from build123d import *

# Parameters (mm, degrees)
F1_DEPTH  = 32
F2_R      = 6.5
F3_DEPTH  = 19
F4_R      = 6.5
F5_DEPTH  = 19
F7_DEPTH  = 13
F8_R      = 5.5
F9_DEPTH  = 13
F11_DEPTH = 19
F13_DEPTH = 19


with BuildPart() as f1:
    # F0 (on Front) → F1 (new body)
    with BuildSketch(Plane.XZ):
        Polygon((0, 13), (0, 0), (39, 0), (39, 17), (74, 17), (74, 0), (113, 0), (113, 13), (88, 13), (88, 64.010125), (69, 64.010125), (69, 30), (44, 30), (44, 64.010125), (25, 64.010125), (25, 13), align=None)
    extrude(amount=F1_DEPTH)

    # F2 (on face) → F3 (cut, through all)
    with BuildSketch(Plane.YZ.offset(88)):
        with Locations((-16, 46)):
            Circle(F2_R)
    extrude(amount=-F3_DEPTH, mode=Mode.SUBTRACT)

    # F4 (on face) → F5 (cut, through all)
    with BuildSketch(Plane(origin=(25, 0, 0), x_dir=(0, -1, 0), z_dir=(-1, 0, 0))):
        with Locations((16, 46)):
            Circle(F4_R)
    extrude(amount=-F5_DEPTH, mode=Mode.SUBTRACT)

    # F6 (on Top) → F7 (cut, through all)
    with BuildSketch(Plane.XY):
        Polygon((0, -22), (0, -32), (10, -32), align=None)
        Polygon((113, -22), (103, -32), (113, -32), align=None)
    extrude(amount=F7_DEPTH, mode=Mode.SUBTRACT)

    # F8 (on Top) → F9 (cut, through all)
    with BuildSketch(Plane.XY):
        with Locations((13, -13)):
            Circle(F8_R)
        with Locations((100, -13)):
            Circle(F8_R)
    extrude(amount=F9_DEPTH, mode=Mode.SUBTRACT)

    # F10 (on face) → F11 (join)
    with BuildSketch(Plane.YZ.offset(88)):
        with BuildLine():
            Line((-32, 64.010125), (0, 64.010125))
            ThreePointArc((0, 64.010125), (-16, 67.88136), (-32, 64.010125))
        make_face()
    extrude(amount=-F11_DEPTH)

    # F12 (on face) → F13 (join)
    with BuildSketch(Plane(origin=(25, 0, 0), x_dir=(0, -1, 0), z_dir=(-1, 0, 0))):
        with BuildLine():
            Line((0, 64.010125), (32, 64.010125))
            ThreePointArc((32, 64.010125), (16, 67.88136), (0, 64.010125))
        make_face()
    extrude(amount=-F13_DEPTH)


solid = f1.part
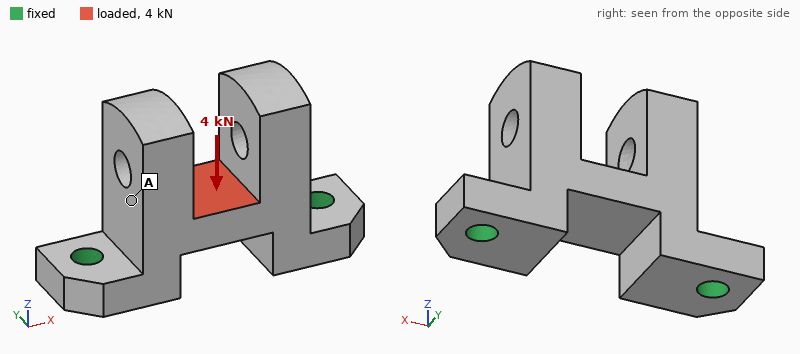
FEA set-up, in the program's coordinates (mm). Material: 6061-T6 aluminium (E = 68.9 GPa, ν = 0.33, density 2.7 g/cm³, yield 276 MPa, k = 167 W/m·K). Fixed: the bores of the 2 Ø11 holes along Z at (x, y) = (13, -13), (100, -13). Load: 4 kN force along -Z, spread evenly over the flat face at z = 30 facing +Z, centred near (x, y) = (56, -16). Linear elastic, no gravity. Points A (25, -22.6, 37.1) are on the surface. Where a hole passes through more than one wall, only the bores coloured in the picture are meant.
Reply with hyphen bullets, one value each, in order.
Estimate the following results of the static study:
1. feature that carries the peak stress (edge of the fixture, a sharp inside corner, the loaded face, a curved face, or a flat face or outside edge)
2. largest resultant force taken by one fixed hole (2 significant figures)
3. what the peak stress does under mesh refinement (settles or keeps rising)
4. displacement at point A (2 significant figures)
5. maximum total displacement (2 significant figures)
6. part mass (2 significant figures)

- edge of the fixture
- 3.0 kN
- keeps rising
- 8.4 µm
- 22 µm
- 260 g
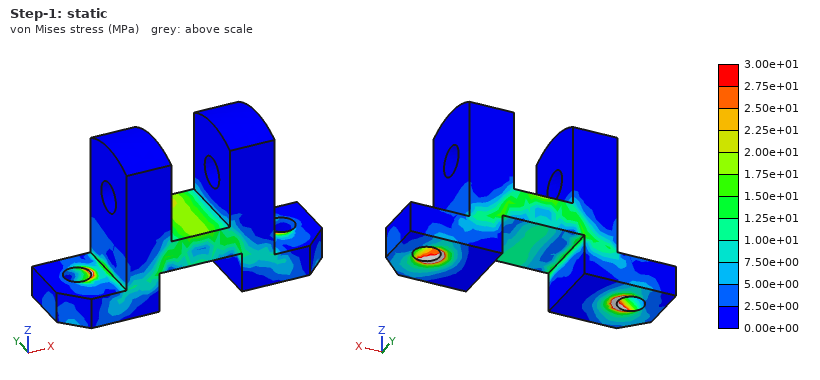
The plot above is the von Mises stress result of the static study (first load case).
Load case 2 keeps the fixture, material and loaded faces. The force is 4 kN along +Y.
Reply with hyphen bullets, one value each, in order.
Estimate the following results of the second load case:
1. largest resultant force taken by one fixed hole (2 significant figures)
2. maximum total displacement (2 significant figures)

- 2.0 kN
- 91 µm
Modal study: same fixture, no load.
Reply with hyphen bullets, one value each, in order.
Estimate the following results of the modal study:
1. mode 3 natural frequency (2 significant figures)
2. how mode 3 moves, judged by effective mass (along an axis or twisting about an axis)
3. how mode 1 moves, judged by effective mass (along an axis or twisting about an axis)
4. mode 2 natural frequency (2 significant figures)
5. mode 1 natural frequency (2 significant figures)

- 4900 Hz
- along X
- along Y
- 4100 Hz
- 2500 Hz
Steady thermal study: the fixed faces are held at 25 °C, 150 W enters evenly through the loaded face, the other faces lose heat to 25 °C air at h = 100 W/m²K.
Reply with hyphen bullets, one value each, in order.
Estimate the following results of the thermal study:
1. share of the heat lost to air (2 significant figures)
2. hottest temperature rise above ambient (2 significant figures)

- 24 %
- 40 K
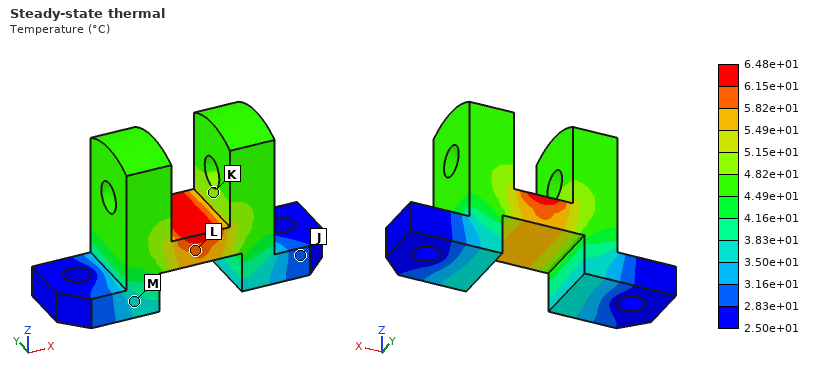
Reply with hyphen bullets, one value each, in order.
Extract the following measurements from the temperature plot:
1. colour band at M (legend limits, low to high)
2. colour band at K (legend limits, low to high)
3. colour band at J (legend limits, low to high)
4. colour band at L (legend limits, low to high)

- 3.50e+01 to 3.83e+01 °C
- 4.82e+01 to 5.15e+01 °C
- 2.83e+01 to 3.16e+01 °C
- 5.82e+01 to 6.15e+01 °C
